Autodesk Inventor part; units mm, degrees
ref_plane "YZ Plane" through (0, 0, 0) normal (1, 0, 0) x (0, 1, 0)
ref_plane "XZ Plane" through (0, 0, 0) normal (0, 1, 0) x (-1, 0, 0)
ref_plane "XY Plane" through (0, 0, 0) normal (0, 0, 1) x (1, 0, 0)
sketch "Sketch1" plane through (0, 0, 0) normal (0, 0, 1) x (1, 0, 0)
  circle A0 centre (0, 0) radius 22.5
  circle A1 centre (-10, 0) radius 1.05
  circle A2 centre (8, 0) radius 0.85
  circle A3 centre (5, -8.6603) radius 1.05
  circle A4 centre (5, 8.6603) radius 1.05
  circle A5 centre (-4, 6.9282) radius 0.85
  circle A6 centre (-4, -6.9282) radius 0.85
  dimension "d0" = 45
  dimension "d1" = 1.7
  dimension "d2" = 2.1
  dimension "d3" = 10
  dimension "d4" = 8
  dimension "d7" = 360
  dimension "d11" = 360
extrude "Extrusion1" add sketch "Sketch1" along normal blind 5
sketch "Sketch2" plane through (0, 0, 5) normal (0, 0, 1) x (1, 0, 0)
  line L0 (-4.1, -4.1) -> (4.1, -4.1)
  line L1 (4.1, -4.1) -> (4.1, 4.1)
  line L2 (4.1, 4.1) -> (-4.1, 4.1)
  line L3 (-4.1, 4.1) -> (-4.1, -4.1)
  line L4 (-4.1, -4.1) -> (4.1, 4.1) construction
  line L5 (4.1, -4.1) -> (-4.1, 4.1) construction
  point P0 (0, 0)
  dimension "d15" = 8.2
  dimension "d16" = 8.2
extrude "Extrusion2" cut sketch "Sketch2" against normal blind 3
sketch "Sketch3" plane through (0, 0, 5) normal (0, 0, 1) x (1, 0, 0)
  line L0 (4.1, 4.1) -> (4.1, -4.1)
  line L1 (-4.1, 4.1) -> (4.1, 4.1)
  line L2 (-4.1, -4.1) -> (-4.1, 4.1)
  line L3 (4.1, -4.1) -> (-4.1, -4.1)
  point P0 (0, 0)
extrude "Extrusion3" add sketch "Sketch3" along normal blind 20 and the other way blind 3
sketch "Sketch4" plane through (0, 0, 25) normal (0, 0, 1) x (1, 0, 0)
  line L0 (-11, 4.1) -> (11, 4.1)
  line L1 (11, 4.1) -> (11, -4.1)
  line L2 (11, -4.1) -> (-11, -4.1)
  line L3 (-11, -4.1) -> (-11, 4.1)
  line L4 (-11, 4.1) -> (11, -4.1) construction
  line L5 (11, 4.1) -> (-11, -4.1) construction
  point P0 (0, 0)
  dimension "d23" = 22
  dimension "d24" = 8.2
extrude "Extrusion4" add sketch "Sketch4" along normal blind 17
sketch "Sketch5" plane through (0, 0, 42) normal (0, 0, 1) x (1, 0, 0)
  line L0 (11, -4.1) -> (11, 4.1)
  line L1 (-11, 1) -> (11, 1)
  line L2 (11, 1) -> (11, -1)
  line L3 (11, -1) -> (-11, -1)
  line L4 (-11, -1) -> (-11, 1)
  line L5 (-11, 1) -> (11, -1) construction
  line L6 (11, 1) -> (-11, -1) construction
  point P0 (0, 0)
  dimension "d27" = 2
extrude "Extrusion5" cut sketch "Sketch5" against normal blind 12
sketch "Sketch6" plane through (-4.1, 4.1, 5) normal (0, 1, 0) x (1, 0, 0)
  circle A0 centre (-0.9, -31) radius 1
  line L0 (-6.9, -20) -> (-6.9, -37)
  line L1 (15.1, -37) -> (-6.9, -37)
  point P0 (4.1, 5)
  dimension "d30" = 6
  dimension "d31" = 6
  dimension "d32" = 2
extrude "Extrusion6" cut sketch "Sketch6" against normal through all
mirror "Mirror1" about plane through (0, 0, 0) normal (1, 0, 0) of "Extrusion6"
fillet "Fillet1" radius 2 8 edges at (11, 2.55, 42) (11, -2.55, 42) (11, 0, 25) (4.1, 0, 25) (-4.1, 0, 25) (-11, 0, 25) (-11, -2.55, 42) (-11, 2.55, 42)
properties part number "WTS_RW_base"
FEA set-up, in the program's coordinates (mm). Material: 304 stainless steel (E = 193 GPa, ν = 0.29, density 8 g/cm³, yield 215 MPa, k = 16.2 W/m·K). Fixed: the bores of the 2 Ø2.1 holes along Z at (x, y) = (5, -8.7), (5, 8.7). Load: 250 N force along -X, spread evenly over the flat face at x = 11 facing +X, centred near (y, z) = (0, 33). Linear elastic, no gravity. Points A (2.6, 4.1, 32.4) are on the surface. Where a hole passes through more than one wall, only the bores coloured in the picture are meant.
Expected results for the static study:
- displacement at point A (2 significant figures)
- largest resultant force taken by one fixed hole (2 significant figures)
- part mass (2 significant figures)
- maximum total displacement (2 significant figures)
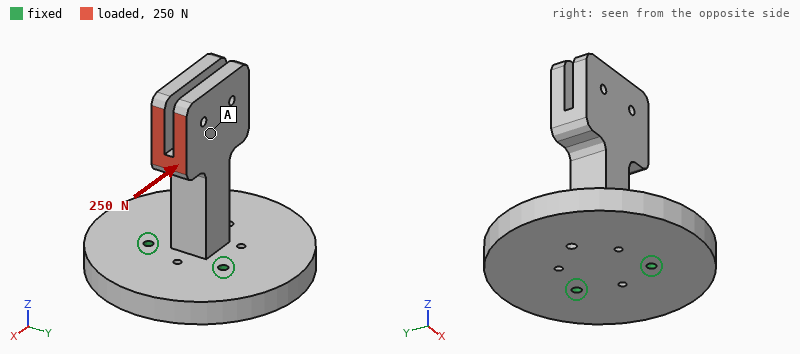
54 µm
130 N
94 g
79 µm
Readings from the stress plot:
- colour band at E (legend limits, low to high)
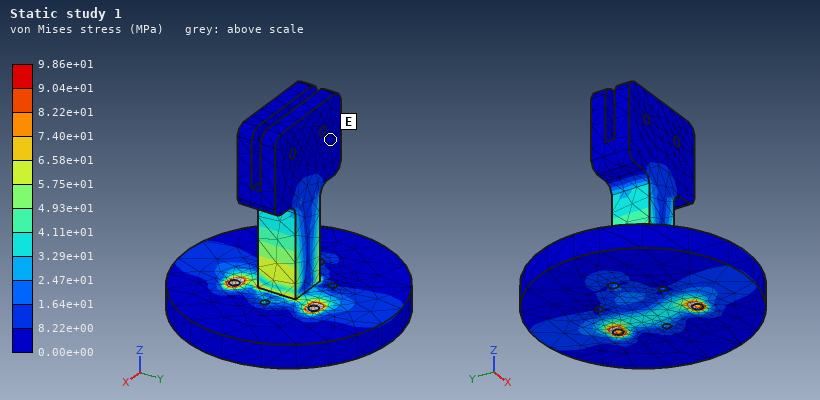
0.00e+00 to 8.22e+00 MPa
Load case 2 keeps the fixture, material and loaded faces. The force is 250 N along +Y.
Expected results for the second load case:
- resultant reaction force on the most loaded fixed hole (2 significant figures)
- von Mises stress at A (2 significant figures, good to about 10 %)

490 N
16 MPa
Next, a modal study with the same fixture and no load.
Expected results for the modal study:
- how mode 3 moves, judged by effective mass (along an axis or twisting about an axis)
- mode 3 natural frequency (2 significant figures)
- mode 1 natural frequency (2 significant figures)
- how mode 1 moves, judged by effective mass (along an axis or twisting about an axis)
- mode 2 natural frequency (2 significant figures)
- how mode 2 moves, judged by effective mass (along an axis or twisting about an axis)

along Z
6300 Hz
2200 Hz
along X
2700 Hz
along Y
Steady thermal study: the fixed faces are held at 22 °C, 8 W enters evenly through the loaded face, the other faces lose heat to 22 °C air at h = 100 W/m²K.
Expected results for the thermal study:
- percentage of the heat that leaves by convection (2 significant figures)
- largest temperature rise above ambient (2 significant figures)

92 %
70 K
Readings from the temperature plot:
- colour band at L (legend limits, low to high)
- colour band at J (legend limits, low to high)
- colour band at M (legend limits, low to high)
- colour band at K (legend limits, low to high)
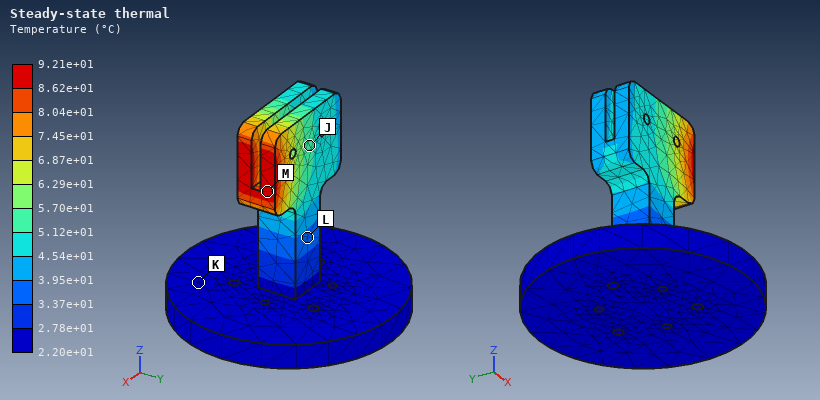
3.37e+01 to 3.95e+01 °C
5.12e+01 to 5.70e+01 °C
8.62e+01 to 9.21e+01 °C
2.20e+01 to 2.78e+01 °C
